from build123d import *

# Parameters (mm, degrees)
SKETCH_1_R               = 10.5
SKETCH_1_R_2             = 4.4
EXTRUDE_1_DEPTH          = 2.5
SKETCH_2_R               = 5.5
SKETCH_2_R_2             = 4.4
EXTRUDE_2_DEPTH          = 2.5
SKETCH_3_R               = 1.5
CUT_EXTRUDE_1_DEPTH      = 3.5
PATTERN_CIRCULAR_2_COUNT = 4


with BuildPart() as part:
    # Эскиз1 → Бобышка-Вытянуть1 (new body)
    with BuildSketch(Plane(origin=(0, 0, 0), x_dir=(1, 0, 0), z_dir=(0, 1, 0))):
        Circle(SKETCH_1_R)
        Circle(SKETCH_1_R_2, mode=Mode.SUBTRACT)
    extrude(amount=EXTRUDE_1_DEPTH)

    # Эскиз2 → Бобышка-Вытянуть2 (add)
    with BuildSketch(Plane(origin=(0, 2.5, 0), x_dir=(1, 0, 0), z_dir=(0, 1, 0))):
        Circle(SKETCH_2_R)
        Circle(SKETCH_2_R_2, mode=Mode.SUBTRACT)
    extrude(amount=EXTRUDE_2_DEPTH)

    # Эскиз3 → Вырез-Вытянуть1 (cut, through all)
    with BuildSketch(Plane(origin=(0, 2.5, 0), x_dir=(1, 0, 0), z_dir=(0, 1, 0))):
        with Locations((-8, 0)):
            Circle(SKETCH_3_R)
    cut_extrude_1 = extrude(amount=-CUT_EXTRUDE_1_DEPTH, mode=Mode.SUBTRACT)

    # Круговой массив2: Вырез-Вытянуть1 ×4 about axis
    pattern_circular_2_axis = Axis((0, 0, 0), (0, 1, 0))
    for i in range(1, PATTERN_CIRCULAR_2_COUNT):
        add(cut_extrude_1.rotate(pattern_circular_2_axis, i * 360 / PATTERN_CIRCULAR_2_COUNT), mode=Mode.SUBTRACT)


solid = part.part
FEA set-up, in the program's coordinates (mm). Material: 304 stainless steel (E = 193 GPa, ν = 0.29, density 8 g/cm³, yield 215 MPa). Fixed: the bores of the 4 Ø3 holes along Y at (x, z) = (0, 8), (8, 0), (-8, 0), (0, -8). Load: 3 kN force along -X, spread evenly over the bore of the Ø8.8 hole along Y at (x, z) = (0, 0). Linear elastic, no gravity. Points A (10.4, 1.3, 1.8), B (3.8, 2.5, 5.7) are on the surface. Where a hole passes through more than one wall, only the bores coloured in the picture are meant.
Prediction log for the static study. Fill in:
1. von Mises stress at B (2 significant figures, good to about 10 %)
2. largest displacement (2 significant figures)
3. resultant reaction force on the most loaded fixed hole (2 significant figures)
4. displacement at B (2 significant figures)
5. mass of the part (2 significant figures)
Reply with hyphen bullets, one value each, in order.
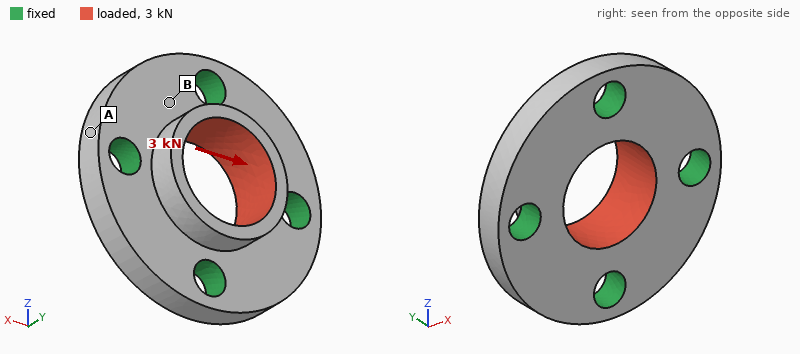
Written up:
- 30 MPa
- 4.8 µm
- 820 N
- 0.97 µm
- 5.8 g
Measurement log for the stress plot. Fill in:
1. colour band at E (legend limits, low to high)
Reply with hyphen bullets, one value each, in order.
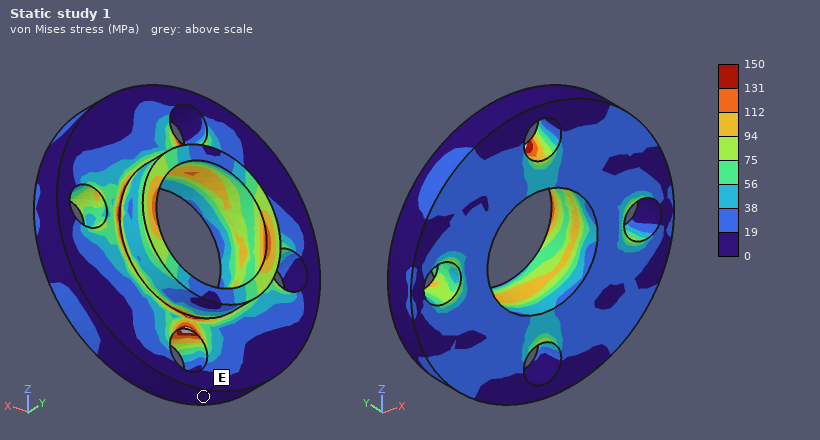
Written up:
- 0 to 19 MPa
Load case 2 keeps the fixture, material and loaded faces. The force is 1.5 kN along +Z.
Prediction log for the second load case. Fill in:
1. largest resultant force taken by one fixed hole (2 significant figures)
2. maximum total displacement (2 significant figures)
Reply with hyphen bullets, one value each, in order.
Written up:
- 410 N
- 2.4 µm
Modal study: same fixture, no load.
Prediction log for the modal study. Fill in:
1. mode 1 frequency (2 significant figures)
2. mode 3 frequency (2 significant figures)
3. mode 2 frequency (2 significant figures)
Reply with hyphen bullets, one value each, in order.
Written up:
- 75 kHz
- 77 kHz
- 77 kHz
